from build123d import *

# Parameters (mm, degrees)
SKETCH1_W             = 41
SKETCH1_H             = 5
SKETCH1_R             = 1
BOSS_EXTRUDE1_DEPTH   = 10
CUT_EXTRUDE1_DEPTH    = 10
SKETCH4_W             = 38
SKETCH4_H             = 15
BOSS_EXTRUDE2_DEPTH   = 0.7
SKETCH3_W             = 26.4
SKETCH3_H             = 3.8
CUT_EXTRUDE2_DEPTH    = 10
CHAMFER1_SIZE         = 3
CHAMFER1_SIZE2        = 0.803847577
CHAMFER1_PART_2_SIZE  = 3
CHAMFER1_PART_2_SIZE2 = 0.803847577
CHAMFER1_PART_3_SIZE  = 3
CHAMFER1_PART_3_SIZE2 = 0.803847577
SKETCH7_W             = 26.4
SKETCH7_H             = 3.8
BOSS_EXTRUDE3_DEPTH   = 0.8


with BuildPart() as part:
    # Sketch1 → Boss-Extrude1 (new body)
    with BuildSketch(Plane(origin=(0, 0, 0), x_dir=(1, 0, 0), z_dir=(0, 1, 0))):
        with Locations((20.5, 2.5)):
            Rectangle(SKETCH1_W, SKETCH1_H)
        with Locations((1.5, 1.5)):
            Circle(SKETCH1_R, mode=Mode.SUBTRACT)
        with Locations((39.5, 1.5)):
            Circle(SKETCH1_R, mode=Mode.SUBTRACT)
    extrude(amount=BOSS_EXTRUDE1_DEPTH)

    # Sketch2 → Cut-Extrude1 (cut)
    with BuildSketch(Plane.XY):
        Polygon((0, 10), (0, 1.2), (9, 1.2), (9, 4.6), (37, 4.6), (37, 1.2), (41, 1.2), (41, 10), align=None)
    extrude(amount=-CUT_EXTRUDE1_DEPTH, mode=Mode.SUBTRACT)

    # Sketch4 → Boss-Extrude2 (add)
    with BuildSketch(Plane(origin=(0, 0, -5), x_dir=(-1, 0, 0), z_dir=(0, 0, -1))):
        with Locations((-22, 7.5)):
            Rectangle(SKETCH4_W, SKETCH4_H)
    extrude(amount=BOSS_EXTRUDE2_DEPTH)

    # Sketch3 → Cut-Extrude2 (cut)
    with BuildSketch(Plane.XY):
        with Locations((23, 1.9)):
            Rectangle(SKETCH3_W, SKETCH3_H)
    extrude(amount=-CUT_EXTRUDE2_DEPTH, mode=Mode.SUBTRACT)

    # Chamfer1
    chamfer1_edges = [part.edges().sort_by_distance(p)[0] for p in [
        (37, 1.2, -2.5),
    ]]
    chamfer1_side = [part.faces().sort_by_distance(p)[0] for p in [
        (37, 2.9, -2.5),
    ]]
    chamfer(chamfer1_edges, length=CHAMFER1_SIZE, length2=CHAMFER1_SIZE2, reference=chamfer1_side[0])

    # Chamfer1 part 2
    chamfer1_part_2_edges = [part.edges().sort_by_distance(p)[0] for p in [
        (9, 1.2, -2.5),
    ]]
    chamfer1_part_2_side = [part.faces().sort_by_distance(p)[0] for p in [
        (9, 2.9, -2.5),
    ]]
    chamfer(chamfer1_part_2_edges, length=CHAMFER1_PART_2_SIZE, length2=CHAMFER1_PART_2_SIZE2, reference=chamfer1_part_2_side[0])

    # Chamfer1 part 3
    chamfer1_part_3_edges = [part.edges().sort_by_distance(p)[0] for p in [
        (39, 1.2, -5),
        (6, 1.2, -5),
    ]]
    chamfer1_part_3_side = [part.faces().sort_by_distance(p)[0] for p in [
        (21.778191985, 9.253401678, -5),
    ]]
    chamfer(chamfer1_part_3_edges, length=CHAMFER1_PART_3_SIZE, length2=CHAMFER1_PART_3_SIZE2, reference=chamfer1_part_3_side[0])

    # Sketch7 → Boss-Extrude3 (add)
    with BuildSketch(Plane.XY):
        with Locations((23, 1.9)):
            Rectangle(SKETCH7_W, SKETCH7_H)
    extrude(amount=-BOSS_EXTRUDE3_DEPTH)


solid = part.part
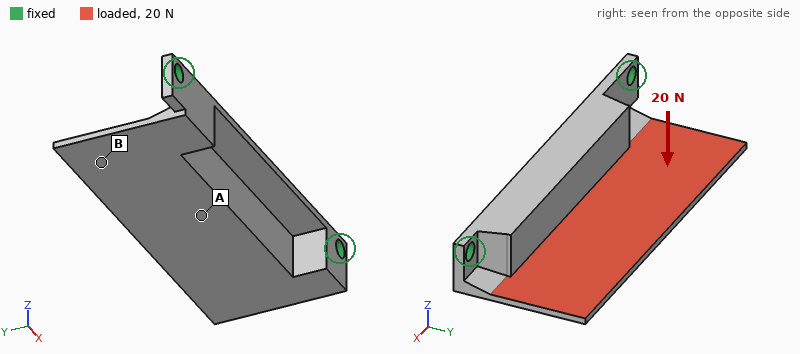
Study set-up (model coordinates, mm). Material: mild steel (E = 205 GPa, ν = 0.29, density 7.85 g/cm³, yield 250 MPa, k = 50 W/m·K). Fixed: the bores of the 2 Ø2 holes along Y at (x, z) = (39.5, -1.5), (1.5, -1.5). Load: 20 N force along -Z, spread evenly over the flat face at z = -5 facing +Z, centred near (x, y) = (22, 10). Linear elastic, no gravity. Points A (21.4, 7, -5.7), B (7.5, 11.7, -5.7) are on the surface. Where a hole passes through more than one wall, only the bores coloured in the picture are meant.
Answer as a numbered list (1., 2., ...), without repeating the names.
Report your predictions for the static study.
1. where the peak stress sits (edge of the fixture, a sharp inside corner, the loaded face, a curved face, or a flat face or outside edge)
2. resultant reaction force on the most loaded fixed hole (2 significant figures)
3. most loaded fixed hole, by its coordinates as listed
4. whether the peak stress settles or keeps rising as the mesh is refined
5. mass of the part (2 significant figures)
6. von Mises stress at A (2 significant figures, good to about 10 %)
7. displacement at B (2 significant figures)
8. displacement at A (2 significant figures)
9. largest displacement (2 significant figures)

1. edge of the fixture
2. 15 N
3. (39.5, -1.5)
4. keeps rising
5. 5.1 g
6. 16 MPa
7. 25 µm
8. 10 µm
9. 35 µm
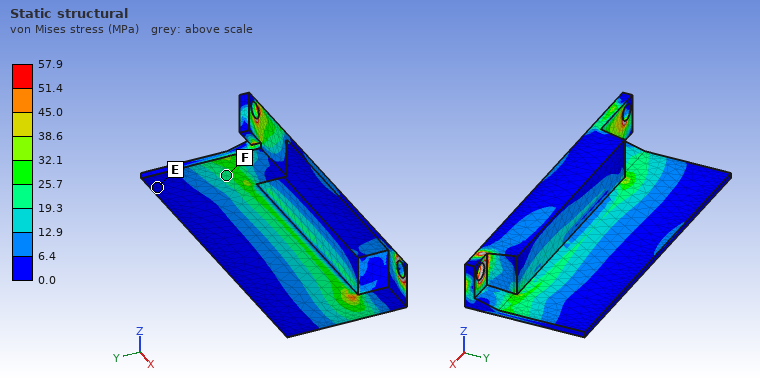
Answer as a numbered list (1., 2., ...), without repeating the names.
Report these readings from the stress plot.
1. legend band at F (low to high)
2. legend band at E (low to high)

1. 19.3 to 25.7 MPa
2. 0.0 to 6.4 MPa
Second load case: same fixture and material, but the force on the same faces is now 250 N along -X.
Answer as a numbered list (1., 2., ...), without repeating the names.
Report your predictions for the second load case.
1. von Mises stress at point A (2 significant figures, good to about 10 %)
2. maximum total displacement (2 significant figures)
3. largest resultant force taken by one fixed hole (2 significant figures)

1. 13 MPa
2. 16 µm
3. 150 N
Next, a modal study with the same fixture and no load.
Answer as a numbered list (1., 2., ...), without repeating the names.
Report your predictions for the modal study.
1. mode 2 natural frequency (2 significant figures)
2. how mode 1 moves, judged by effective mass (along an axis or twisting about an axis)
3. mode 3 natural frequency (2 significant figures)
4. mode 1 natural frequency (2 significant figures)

1. 5000 Hz
2. along Z
3. 7700 Hz
4. 3200 Hz
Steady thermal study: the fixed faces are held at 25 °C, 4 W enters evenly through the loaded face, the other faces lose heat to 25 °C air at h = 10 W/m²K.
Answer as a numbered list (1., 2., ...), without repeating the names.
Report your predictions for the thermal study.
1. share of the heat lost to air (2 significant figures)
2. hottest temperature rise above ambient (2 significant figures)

1. 11 %
2. 54 K
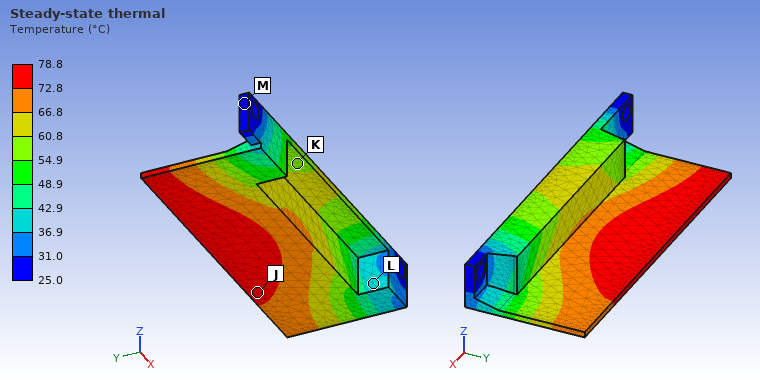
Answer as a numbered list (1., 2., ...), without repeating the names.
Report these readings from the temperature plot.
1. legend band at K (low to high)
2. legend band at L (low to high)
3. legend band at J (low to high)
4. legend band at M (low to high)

1. 54.9 to 60.8 °C
2. 36.9 to 42.9 °C
3. 72.8 to 78.8 °C
4. 25.0 to 31.0 °C
